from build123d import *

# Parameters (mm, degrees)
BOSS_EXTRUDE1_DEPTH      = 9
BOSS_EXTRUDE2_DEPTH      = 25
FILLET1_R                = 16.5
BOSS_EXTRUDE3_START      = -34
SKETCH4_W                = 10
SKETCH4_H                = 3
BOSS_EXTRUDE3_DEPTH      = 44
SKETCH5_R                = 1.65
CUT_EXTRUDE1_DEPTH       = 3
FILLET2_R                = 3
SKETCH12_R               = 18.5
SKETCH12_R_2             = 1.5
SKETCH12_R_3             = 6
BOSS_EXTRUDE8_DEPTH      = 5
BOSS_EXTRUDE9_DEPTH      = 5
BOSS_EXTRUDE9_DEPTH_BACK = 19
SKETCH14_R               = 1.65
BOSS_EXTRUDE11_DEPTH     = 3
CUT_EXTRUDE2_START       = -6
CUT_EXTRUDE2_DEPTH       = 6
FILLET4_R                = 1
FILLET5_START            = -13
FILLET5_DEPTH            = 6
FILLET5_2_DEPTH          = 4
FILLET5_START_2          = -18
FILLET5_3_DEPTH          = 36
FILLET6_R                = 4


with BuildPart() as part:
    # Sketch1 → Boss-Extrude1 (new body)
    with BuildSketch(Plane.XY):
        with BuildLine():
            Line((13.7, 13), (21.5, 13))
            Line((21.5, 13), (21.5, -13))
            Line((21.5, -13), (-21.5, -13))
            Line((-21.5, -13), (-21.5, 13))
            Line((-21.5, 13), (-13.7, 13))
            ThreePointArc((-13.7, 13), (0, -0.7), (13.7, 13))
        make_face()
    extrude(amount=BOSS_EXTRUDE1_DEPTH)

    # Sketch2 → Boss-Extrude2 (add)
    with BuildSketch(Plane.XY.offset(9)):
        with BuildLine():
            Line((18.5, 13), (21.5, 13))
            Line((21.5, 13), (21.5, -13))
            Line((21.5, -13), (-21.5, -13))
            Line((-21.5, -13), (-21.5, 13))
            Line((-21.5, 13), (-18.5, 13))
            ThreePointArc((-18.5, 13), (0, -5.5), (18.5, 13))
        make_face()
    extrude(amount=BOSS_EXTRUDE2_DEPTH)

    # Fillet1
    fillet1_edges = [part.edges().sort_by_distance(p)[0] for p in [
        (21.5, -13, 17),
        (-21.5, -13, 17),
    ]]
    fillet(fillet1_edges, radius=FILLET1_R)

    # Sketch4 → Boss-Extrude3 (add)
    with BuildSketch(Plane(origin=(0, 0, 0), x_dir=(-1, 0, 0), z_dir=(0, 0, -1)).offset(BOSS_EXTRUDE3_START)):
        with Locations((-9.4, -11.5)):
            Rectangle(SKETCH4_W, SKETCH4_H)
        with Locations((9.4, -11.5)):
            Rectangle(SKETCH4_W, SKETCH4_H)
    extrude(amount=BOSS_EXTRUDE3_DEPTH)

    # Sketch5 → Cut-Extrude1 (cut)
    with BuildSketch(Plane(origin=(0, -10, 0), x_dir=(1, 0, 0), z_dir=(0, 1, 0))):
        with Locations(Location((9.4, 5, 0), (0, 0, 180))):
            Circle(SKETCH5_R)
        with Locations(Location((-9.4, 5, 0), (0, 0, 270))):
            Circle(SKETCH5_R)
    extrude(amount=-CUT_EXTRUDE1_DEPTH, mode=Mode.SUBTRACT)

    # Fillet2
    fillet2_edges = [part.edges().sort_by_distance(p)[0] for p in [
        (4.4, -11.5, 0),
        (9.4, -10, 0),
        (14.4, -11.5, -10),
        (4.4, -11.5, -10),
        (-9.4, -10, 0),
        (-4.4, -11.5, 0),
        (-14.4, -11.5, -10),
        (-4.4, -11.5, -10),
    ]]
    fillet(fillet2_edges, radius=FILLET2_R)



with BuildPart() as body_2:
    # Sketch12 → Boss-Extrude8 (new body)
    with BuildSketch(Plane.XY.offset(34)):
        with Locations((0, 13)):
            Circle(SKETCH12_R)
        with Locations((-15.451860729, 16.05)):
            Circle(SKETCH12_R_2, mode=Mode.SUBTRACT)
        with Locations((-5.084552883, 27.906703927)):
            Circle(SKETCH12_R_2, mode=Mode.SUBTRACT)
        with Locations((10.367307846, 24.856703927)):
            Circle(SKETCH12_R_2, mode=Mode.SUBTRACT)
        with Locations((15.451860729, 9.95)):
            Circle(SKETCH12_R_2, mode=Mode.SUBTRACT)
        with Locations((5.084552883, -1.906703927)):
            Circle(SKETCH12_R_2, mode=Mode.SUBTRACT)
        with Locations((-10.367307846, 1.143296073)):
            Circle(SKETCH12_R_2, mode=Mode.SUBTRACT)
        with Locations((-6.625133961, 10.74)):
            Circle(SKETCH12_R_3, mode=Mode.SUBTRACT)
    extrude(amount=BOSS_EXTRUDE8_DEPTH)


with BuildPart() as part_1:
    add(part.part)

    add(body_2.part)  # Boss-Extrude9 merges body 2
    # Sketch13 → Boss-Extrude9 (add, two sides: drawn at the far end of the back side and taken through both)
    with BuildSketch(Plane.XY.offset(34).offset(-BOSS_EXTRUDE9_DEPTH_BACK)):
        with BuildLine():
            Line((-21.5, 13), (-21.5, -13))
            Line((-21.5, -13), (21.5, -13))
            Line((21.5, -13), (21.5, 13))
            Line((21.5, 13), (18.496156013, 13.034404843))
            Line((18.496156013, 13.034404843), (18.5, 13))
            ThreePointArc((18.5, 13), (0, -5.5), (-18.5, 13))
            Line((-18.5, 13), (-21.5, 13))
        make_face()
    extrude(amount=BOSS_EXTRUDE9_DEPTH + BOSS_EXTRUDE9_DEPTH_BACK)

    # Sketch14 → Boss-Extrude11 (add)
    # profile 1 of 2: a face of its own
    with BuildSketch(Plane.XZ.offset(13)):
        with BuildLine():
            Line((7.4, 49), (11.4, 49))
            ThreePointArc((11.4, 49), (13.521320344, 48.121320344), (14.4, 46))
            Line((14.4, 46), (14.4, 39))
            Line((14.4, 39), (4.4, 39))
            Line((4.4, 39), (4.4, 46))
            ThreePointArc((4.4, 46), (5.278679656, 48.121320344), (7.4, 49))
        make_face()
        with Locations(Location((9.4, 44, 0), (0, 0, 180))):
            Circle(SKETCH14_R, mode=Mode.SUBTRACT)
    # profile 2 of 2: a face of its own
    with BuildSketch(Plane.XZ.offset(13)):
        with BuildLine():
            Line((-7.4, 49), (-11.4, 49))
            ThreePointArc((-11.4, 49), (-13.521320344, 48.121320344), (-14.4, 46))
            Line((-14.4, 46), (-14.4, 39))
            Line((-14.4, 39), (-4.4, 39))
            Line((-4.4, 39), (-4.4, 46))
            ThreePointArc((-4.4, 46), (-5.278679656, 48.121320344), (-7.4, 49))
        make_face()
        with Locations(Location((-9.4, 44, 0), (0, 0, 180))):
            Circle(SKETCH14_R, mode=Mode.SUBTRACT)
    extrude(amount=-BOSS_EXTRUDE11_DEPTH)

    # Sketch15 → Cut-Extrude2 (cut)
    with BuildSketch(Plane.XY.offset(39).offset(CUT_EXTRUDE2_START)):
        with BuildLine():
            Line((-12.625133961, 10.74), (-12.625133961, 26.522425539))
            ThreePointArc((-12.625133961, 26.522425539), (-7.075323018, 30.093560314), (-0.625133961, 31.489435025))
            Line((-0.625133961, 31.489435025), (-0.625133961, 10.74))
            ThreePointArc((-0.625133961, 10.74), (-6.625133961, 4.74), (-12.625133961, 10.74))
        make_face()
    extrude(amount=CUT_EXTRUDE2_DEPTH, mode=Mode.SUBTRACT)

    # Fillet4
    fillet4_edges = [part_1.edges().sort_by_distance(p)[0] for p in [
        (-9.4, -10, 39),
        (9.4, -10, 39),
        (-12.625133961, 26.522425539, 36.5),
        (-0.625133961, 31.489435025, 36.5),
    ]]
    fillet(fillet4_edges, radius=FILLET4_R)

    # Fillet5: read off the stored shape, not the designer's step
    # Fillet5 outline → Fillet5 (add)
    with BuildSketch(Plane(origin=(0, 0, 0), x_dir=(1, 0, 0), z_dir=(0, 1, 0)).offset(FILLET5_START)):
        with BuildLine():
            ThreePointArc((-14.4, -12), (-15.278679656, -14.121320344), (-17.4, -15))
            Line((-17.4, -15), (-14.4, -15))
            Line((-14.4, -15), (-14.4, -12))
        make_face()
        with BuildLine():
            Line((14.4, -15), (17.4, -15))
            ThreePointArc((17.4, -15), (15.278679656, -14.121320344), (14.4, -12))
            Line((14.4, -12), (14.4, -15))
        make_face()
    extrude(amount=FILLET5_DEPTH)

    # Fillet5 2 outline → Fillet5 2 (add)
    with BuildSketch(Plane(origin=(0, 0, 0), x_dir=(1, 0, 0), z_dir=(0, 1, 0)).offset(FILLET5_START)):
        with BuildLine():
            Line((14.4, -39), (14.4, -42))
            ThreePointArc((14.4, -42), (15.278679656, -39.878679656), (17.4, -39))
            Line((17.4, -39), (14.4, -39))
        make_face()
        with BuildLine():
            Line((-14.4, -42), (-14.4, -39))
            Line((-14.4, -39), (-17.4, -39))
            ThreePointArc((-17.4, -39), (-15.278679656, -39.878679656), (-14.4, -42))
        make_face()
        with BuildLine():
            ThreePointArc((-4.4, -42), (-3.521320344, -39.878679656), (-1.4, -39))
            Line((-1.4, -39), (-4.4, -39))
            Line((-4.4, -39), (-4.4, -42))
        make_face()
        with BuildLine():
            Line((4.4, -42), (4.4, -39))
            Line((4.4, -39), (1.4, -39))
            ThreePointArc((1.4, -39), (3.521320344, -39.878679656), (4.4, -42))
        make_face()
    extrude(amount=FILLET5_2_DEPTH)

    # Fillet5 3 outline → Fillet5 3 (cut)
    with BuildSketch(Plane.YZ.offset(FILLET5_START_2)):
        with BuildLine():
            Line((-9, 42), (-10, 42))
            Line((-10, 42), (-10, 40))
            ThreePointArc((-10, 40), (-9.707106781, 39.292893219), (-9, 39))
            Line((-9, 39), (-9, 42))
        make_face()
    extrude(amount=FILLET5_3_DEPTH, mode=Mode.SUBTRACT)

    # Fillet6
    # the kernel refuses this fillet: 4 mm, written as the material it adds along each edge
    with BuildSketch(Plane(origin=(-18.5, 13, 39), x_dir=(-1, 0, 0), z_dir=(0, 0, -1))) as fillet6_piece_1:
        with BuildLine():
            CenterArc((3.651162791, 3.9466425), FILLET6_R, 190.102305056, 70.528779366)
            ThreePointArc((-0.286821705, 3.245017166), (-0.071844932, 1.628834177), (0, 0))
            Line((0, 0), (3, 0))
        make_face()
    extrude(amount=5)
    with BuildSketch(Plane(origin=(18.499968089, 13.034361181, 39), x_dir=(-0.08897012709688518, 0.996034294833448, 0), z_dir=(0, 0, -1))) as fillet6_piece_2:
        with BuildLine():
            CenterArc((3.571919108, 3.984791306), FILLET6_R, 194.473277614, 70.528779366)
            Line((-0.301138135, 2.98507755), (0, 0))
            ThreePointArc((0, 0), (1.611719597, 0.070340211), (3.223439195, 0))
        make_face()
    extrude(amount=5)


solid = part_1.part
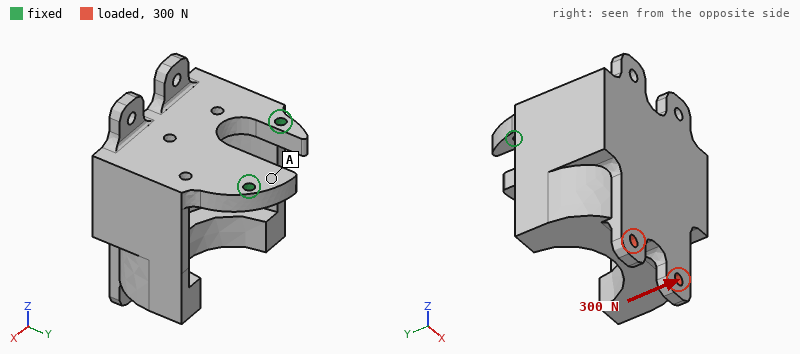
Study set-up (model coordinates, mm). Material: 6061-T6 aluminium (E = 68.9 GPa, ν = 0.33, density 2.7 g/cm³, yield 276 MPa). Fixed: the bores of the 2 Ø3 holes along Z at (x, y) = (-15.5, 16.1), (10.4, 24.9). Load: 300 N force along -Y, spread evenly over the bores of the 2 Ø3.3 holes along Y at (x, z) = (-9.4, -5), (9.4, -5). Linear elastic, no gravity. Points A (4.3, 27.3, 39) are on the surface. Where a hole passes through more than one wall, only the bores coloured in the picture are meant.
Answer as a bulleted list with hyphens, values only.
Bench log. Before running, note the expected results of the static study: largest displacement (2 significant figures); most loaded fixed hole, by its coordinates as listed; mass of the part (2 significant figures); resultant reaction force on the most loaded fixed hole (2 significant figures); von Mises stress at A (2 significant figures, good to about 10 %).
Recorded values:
- 0.53 mm
- (10.4, 24.9)
- 76 g
- 190 N
- 22 MPa
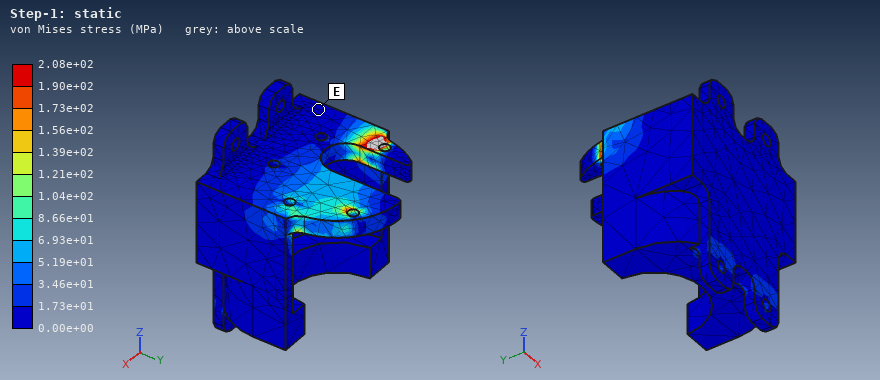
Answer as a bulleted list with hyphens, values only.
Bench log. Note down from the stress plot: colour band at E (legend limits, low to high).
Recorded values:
- 0.00e+00 to 1.73e+01 MPa
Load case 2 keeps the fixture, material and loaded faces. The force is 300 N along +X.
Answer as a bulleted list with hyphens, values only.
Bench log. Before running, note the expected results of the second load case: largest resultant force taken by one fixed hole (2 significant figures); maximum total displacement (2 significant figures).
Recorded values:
- 480 N
- 0.12 mm
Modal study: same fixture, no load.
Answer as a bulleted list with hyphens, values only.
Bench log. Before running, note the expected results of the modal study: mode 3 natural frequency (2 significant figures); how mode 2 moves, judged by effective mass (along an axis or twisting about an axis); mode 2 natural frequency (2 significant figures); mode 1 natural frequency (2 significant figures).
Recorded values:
- 4800 Hz
- along X
- 1900 Hz
- 760 Hz
